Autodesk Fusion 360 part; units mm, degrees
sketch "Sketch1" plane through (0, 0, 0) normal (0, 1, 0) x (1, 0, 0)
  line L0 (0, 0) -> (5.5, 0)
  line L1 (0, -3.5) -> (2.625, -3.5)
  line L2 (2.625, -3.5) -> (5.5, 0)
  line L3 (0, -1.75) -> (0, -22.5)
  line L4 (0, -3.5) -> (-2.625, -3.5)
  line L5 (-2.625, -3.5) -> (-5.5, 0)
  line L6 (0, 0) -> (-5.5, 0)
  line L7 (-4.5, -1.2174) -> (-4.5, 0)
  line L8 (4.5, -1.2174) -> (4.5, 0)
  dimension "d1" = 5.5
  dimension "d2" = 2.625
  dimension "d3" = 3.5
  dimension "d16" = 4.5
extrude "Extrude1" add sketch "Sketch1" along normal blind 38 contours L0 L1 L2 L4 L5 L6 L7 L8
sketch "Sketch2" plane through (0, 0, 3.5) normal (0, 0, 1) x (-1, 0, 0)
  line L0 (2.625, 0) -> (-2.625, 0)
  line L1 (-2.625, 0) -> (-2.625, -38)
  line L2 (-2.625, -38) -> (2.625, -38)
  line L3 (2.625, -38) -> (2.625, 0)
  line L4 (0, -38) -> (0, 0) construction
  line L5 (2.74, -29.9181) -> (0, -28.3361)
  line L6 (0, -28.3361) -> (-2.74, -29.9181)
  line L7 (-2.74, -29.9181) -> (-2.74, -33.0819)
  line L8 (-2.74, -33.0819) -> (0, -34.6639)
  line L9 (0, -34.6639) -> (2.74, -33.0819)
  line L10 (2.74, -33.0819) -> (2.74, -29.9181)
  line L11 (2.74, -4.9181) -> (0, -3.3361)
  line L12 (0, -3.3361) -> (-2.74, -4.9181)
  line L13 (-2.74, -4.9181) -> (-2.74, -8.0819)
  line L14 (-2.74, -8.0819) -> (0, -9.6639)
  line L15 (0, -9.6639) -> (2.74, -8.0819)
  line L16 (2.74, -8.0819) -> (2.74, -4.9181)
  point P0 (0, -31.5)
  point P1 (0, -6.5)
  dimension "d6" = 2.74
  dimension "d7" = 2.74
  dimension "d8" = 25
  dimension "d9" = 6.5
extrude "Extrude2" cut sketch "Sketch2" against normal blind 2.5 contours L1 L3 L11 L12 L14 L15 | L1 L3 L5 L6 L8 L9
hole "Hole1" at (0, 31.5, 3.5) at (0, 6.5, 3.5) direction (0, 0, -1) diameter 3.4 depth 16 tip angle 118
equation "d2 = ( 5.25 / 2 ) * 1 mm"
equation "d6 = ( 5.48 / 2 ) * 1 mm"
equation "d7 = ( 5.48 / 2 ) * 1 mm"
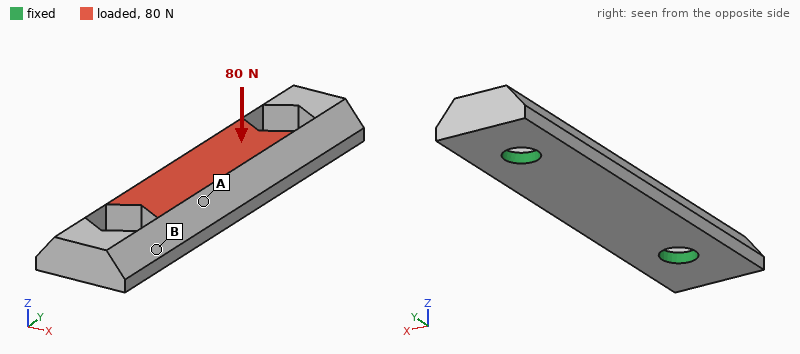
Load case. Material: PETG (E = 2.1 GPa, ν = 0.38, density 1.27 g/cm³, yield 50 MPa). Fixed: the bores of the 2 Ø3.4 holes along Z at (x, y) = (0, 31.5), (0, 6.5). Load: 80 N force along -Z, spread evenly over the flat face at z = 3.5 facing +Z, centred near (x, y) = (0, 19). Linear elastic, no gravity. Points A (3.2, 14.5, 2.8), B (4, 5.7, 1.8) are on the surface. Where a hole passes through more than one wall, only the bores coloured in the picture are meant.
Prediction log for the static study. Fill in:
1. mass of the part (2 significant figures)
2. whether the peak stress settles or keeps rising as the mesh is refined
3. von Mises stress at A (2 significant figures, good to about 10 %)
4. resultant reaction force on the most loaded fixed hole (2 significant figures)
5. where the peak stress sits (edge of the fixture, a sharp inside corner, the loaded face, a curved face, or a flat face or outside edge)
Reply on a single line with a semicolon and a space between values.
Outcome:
1.1 g; keeps rising; 6.4 MPa; 63 N; edge of the fixture
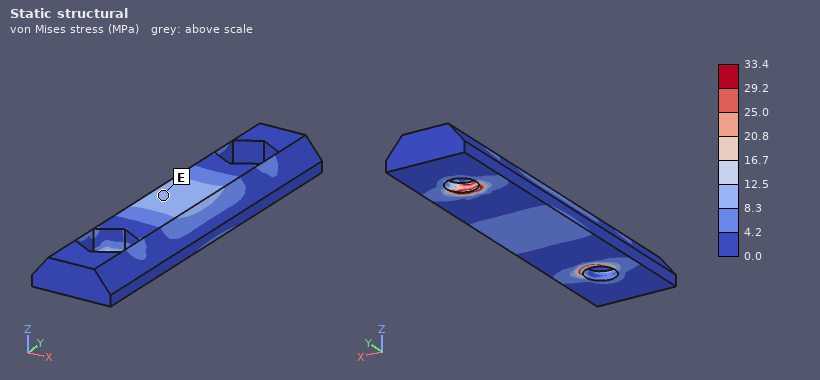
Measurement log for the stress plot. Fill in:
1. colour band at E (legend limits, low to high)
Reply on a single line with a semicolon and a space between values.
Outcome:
8.3 to 12.5 MPa
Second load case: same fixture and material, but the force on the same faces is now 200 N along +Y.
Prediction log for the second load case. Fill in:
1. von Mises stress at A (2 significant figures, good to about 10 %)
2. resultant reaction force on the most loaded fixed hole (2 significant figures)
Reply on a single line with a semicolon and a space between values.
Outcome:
2.8 MPa; 100 N
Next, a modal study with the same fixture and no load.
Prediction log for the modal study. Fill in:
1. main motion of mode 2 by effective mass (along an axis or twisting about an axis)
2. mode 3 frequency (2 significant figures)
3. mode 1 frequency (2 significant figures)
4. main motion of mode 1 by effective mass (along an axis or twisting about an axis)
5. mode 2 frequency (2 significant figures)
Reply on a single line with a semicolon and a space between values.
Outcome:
along X; 7700 Hz; 5000 Hz; along Z; 6200 Hz
